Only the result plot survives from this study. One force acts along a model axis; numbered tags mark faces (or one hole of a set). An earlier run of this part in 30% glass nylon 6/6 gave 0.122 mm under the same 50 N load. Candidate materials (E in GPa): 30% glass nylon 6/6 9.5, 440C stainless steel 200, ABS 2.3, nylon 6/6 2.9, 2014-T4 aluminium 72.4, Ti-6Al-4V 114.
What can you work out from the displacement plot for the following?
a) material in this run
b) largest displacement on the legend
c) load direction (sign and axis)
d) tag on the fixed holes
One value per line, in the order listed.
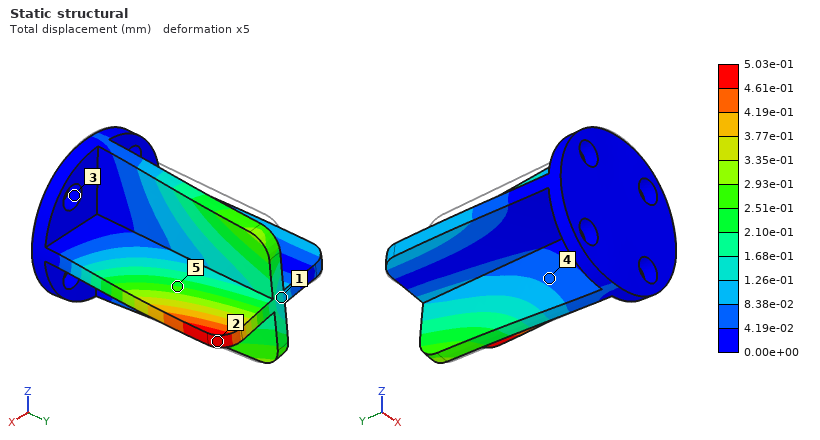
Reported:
ABS
5.03e-01 mm
-Z
3
